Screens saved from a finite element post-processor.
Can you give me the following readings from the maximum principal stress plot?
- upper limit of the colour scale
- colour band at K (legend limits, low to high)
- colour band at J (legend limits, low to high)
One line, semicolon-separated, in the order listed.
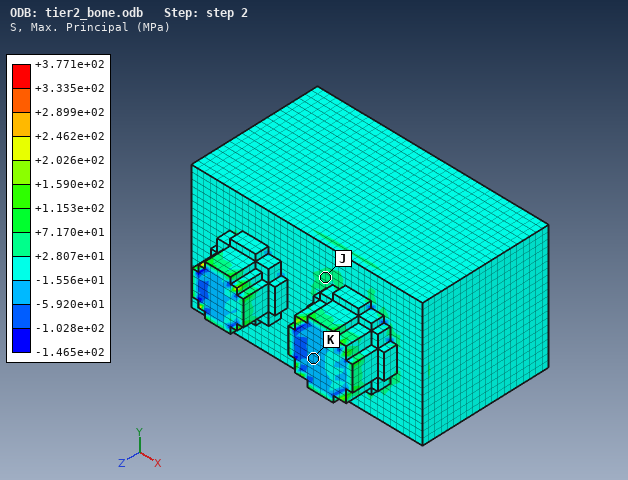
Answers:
+3.771e+02 MPa; -5.920e+01 to -1.556e+01 MPa; +2.807e+01 to +7.170e+01 MPa
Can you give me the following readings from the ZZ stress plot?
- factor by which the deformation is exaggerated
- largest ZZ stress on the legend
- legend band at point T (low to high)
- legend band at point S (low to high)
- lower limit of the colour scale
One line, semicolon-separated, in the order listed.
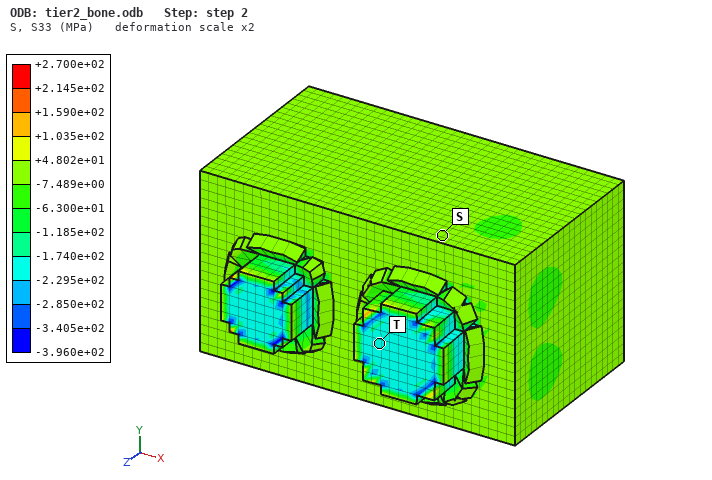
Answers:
2; +2.700e+02 MPa; -2.295e+02 to -1.740e+02 MPa; -7.489e+00 to +4.802e+01 MPa; -3.960e+02 MPa
